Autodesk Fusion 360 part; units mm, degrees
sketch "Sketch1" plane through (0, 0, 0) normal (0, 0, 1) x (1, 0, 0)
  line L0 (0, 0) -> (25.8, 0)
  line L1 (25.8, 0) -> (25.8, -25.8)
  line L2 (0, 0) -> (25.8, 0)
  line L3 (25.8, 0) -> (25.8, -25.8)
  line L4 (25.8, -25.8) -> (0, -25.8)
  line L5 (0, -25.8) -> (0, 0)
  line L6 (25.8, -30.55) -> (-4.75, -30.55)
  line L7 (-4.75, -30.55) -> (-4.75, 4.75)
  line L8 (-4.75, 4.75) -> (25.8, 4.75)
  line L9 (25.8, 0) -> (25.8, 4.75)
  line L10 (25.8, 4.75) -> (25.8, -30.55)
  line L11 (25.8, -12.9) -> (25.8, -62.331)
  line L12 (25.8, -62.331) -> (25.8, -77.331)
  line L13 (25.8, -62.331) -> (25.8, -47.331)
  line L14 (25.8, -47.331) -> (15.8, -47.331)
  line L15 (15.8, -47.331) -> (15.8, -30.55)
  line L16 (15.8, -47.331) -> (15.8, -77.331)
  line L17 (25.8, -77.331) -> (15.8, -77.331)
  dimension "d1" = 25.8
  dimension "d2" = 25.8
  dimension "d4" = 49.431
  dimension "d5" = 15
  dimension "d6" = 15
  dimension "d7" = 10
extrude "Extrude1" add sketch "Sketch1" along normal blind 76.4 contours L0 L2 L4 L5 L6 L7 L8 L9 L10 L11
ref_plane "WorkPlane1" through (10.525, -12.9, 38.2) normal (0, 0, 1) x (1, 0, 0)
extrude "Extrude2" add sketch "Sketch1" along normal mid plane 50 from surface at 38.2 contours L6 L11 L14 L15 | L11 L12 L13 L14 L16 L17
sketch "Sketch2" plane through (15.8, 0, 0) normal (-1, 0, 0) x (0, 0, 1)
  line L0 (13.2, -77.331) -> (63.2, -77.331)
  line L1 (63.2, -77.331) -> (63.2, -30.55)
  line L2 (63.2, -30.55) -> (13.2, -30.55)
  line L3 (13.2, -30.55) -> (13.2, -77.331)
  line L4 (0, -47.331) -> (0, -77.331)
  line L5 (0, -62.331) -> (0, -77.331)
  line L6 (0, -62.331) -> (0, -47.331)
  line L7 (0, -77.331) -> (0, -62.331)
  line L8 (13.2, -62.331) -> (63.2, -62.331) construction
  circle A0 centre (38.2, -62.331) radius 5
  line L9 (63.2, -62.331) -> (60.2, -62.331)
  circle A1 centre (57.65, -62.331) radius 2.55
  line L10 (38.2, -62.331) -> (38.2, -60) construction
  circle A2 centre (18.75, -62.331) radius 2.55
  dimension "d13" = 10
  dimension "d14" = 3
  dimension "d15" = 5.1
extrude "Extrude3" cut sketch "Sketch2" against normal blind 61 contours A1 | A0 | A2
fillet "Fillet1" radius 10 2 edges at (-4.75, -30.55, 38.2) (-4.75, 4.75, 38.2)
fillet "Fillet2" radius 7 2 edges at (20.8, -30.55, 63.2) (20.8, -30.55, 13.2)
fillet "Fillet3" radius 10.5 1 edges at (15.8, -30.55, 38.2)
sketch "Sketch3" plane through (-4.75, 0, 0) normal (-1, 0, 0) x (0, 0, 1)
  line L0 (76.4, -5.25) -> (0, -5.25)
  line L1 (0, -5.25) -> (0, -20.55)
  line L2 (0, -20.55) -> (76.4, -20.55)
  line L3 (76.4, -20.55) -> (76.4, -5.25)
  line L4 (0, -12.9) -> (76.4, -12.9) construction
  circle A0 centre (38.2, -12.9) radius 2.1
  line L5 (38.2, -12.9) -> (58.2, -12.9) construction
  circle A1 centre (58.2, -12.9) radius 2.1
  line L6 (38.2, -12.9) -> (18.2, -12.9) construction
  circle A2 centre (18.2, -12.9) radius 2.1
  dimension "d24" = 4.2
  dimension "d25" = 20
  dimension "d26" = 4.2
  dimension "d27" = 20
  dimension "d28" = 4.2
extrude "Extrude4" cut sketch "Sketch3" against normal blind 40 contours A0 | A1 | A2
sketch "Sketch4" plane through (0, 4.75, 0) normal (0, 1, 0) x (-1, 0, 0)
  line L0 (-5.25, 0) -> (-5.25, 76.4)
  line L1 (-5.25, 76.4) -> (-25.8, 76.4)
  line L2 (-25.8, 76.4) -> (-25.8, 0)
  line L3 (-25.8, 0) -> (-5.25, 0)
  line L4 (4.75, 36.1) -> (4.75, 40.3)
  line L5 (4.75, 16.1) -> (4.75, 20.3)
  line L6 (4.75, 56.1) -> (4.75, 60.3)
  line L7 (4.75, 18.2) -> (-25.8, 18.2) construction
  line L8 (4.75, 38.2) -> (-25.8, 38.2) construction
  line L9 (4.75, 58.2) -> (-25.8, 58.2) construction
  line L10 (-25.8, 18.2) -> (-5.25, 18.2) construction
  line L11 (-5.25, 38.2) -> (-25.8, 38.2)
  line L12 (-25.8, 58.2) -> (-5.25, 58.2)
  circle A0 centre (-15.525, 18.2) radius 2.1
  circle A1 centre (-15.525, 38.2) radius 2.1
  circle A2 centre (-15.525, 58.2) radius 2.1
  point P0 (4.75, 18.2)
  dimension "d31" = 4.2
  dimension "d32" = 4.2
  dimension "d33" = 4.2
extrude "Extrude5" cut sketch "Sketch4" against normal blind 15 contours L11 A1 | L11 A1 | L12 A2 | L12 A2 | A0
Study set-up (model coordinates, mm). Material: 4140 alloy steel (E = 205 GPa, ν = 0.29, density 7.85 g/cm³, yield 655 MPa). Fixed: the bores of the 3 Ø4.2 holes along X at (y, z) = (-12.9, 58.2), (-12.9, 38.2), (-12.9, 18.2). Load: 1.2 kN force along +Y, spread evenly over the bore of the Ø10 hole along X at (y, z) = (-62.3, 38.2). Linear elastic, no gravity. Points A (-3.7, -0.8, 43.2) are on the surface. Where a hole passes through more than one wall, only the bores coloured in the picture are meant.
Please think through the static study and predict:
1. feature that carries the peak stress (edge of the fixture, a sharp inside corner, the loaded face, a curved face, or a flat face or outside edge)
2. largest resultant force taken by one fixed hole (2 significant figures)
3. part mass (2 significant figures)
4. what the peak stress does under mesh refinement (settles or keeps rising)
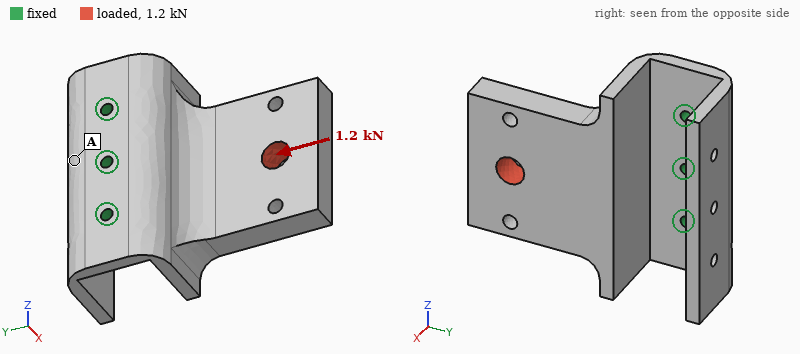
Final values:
edge of the fixture
490 N
400 g
keeps rising
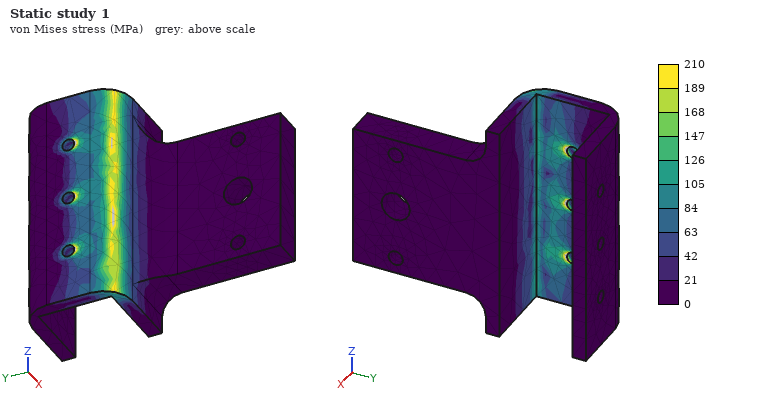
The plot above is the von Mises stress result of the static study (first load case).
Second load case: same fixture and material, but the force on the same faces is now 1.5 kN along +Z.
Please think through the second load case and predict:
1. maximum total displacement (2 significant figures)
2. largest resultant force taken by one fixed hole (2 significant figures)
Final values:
55 µm
2.0 kN
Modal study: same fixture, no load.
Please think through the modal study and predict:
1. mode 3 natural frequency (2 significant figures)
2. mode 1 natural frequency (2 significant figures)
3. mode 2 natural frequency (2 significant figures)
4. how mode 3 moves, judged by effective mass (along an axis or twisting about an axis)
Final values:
2500 Hz
560 Hz
2300 Hz
along Z
